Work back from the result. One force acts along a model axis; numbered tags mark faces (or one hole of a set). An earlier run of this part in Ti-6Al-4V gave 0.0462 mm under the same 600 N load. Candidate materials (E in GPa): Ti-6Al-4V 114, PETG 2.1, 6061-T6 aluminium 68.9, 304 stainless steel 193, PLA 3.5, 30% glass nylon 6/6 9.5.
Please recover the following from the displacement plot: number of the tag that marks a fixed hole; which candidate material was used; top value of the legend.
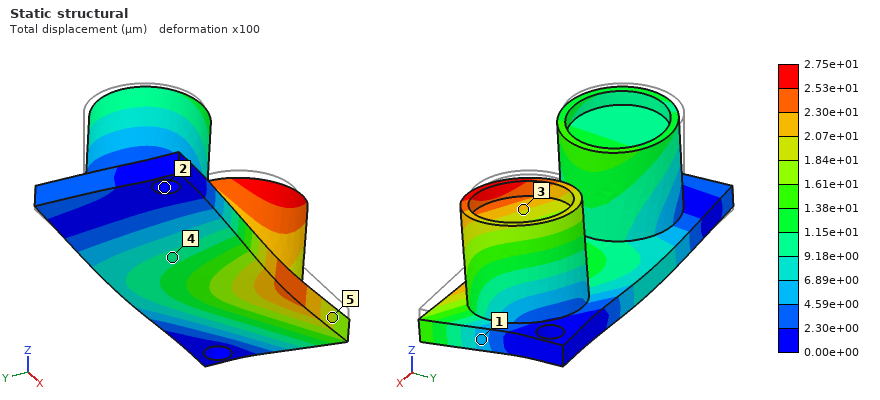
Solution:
2
304 stainless steel
2.75e+01 µm
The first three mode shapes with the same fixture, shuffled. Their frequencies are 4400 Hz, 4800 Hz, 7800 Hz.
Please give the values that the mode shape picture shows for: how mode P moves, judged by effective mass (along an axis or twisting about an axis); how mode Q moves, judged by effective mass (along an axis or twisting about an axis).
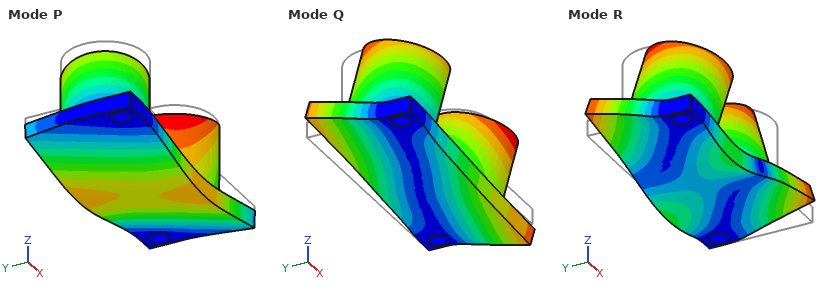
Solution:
along Z
along Y
